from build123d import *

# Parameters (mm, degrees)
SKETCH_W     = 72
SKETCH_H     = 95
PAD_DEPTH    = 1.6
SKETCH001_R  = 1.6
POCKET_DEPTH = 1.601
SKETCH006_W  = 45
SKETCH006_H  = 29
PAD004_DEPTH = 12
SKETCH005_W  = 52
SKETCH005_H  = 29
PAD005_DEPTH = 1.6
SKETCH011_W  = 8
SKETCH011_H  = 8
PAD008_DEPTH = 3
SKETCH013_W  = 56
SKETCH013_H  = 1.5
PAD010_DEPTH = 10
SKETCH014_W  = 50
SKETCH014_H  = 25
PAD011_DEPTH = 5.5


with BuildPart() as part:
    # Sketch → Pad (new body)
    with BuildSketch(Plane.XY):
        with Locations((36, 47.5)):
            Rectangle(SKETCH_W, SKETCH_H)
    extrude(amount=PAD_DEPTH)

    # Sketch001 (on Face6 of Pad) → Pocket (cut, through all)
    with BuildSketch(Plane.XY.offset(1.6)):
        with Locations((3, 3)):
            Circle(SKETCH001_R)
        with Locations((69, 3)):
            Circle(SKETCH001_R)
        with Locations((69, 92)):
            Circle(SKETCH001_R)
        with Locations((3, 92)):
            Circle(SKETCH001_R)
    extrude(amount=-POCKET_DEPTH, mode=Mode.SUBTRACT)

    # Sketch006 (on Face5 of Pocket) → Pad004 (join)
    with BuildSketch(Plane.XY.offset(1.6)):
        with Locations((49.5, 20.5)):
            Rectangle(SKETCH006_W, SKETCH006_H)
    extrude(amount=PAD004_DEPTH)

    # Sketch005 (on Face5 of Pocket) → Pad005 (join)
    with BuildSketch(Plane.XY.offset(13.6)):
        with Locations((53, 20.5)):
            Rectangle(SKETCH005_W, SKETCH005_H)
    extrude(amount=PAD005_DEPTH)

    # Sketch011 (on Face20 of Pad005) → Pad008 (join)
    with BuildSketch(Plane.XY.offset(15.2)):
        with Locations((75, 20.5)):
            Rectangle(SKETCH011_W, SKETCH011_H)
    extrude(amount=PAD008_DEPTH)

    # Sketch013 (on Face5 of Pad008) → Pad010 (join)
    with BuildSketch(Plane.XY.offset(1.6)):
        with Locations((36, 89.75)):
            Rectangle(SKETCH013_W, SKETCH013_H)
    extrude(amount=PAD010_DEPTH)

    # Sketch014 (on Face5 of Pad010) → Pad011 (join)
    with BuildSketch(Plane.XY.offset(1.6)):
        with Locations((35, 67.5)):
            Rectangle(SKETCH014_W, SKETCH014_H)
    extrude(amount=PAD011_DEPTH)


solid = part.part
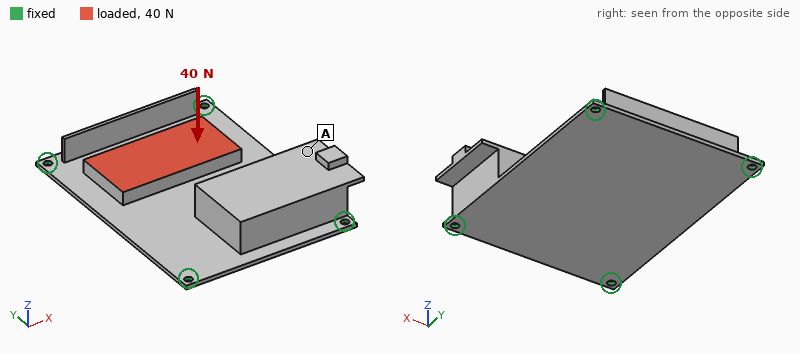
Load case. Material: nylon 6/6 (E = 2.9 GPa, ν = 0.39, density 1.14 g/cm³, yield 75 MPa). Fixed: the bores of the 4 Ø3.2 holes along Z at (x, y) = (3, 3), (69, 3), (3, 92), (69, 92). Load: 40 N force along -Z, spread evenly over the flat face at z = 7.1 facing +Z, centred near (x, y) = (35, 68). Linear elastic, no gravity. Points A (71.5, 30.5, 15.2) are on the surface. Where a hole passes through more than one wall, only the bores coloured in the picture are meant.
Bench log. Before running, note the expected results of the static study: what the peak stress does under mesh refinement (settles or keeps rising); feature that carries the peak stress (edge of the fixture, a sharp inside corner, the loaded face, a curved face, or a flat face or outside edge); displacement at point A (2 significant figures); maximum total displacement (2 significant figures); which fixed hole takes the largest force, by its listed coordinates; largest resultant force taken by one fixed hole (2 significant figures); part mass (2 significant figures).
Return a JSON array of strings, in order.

["keeps rising", "edge of the fixture", "0.91 mm", "1.3 mm", "(3, 92)", "20 N", "42 g"]
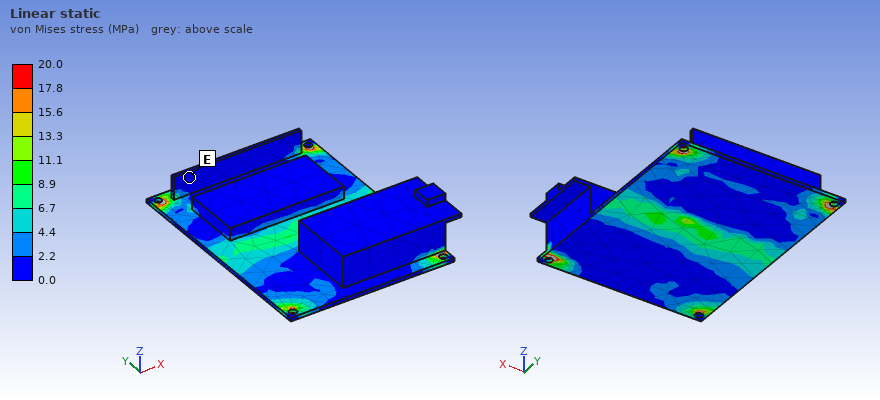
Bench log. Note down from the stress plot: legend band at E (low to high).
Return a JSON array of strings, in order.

["0.0 to 2.2 MPa"]
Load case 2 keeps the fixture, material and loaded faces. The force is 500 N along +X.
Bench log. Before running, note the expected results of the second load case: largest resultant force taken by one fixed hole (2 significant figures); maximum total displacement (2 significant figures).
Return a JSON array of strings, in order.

["220 N", "1.0 mm"]
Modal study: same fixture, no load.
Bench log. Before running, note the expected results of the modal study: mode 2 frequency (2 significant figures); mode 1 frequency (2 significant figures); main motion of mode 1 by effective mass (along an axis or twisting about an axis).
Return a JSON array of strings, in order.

["450 Hz", "180 Hz", "along Z"]
